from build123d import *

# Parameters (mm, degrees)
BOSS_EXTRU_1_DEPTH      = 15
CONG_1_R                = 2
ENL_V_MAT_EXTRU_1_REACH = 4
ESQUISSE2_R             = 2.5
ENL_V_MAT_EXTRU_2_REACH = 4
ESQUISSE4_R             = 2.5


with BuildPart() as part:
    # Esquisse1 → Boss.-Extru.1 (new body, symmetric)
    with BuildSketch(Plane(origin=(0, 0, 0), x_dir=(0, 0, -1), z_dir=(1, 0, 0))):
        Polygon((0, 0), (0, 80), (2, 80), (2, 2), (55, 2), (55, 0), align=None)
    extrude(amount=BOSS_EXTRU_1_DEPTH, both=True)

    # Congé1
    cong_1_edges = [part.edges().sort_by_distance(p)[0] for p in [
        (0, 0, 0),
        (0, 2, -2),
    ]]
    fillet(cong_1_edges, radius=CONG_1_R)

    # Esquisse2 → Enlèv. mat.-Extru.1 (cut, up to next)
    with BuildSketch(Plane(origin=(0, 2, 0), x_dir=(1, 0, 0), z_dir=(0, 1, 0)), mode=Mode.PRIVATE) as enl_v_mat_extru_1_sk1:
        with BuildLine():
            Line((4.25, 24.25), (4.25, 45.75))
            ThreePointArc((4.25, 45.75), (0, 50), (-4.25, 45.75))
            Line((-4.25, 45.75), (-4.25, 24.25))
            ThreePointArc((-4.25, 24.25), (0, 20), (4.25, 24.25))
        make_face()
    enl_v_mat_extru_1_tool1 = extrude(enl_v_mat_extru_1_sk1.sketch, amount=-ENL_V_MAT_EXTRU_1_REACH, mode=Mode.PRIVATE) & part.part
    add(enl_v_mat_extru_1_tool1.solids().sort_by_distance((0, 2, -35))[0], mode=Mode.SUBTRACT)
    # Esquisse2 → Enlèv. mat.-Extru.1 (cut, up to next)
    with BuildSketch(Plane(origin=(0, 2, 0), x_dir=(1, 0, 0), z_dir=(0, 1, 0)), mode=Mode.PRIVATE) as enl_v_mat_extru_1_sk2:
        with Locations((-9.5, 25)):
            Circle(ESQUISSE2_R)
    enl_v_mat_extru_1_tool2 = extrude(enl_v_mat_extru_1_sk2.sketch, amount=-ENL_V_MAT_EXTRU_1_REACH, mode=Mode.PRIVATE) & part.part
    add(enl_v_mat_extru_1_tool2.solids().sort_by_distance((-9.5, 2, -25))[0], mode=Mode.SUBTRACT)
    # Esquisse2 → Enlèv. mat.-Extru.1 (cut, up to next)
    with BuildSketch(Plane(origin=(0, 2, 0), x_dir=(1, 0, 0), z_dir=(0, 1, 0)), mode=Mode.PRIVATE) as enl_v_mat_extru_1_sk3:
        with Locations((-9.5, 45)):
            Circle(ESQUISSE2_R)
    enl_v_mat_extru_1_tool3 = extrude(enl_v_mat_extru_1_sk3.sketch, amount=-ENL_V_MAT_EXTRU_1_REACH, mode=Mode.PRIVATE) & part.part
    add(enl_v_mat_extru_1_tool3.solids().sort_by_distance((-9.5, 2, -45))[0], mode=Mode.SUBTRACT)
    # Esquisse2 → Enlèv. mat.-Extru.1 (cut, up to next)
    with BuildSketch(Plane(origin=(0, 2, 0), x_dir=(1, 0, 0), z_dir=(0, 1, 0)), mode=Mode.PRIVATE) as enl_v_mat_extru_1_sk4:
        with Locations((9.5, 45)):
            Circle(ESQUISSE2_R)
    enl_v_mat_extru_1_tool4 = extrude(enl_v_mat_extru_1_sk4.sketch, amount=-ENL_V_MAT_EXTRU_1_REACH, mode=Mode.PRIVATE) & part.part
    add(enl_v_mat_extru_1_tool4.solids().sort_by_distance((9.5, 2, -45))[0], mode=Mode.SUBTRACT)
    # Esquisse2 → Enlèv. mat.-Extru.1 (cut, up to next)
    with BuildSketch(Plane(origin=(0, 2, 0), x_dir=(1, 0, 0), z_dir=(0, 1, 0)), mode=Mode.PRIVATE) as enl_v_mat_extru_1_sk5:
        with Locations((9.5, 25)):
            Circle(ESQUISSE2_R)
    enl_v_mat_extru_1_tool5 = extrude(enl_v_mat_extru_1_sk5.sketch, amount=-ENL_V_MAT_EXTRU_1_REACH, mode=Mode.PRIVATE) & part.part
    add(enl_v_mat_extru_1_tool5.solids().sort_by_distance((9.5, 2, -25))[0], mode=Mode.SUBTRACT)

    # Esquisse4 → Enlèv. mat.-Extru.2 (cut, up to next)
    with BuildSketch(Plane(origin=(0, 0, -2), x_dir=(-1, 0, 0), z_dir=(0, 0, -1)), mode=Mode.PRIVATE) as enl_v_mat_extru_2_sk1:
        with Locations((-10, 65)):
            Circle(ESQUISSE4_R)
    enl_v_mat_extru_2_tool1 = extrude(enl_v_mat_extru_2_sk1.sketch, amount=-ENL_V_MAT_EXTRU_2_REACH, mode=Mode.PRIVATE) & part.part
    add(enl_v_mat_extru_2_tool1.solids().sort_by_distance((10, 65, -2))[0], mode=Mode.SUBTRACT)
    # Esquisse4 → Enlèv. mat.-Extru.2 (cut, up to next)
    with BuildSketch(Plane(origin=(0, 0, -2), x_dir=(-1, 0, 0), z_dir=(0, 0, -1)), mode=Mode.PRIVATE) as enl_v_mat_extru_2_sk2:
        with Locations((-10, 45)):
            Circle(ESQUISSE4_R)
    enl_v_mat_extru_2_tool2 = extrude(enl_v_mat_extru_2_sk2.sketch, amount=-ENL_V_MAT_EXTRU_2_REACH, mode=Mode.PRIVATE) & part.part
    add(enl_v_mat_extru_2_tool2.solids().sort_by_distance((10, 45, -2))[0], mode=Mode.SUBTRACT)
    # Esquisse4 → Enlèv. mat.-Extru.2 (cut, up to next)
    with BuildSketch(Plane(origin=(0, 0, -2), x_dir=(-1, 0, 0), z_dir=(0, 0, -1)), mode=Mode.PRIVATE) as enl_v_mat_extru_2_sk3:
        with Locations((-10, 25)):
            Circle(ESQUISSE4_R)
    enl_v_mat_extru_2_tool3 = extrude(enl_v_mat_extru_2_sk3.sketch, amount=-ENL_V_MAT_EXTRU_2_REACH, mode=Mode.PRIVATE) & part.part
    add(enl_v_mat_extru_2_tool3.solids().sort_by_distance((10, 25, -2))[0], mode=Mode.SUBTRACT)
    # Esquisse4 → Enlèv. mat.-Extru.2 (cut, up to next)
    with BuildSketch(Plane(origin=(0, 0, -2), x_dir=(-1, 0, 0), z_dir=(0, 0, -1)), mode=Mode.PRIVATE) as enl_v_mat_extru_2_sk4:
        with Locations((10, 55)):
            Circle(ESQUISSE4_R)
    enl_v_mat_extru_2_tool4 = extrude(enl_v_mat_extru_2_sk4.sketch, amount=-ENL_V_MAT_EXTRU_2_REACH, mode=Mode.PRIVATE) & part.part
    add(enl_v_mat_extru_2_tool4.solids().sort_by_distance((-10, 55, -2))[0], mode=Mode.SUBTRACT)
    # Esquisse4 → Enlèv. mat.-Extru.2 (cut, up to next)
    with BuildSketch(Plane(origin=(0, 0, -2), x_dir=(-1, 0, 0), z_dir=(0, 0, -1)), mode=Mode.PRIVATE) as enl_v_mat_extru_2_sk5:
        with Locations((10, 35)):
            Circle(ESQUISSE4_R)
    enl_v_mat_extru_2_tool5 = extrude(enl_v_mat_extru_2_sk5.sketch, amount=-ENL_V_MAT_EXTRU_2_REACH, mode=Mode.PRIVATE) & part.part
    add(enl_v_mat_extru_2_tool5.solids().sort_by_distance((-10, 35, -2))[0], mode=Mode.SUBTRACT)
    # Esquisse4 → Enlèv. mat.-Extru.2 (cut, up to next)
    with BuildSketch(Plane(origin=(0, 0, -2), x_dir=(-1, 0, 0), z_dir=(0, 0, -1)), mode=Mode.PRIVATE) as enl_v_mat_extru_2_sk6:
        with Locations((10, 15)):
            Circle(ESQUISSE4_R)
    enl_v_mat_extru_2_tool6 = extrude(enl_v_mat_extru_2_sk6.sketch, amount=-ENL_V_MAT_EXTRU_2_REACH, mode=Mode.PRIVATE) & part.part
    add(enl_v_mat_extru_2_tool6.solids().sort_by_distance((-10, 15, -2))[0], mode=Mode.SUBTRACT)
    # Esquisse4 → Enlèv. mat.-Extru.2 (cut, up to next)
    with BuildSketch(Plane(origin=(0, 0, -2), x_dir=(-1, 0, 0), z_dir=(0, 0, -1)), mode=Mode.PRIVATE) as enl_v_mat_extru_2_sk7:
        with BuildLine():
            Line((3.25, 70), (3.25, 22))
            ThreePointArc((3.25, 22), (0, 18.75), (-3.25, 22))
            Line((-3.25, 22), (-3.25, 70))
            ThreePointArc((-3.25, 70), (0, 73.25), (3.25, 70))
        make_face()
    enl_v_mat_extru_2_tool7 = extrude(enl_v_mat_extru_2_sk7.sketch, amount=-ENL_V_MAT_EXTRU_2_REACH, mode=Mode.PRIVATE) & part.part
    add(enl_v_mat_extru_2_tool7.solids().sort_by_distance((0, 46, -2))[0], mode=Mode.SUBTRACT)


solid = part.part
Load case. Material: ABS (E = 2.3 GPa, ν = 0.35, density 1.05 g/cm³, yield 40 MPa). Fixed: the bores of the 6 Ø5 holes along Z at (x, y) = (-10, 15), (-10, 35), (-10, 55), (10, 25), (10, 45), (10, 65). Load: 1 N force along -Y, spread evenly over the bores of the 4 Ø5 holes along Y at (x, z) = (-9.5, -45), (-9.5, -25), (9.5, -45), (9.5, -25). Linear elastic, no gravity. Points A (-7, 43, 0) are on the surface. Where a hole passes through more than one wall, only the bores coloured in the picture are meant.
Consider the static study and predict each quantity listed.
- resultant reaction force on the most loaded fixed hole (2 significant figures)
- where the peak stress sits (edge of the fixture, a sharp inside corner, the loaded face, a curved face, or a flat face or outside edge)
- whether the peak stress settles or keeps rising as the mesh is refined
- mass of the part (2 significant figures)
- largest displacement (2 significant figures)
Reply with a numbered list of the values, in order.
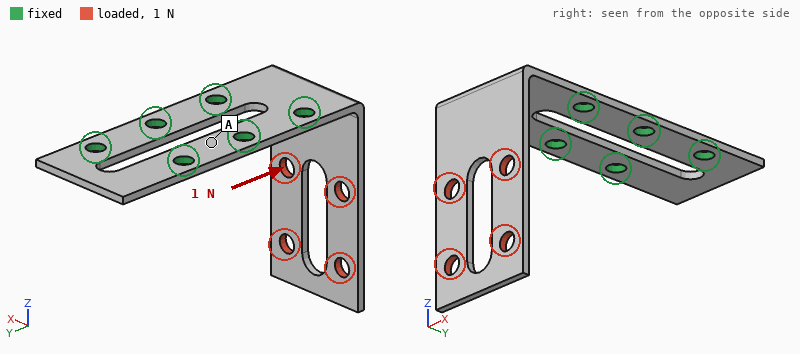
1. 0.79 N
2. edge of the fixture
3. keeps rising
4. 6.7 g
5. 1.1 mm
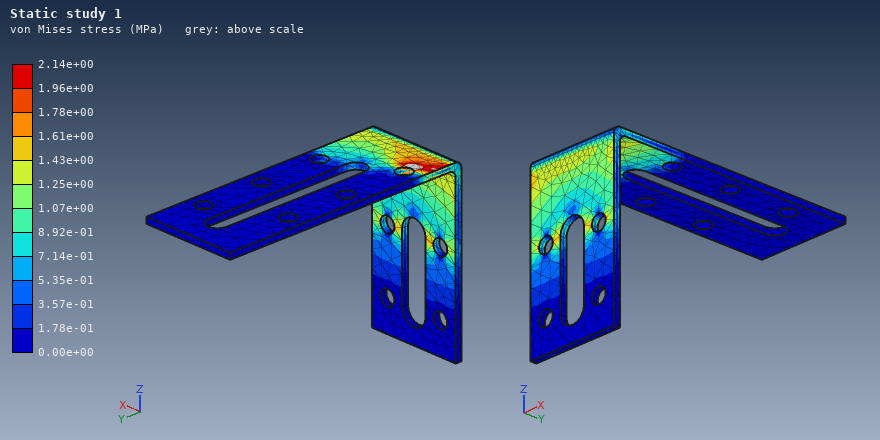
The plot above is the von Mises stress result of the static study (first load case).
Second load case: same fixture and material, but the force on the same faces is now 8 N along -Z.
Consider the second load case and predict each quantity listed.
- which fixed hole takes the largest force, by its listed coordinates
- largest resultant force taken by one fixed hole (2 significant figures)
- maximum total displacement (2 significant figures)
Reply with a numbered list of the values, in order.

1. (-10, 15)
2. 7.1 N
3. 1.2 mm
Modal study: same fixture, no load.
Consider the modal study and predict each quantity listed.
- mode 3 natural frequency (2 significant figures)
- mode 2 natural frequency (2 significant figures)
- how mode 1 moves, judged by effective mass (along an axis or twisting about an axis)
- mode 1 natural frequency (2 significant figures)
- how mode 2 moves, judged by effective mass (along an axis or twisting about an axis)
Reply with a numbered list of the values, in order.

1. 550 Hz
2. 280 Hz
3. along Y
4. 130 Hz
5. along X
